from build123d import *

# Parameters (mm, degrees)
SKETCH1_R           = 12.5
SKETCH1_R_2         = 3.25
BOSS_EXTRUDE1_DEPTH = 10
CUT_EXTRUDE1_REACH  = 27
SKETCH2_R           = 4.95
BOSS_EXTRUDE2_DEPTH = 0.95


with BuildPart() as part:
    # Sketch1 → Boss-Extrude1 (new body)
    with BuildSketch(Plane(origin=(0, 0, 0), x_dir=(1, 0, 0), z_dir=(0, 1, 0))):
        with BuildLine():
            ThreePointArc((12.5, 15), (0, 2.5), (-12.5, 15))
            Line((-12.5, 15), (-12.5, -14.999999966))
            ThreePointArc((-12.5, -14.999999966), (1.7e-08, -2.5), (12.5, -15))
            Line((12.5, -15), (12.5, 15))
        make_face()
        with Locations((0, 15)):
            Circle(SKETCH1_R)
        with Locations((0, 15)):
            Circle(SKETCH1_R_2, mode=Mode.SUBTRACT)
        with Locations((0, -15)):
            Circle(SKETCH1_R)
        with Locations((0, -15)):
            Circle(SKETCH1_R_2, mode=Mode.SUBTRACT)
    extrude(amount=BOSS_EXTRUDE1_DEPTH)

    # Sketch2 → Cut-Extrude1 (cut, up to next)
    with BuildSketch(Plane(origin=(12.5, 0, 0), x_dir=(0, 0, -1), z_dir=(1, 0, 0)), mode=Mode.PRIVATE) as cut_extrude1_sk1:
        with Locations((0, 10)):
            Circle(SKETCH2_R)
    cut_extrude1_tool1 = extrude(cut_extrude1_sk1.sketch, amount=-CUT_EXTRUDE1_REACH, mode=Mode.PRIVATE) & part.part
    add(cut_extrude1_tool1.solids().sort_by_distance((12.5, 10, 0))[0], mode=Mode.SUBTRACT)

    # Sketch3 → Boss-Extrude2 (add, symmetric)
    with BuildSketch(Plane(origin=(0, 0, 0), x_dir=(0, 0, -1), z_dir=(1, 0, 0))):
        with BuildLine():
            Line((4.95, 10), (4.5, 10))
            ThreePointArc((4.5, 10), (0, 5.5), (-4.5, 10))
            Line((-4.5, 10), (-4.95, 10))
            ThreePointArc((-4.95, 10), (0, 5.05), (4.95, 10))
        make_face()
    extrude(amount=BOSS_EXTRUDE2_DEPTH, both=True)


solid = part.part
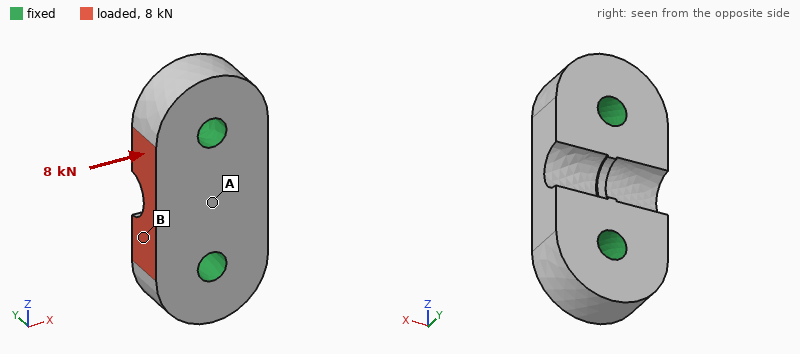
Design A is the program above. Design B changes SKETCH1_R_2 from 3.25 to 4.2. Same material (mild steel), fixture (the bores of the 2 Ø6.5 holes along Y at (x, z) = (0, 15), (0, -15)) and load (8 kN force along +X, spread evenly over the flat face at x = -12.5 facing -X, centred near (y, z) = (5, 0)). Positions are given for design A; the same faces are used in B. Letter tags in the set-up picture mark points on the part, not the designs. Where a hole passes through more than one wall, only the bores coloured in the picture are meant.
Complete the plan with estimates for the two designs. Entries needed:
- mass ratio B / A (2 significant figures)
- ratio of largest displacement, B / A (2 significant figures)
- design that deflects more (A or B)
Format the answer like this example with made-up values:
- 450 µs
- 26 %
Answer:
- 0.96
- 0.86
- A
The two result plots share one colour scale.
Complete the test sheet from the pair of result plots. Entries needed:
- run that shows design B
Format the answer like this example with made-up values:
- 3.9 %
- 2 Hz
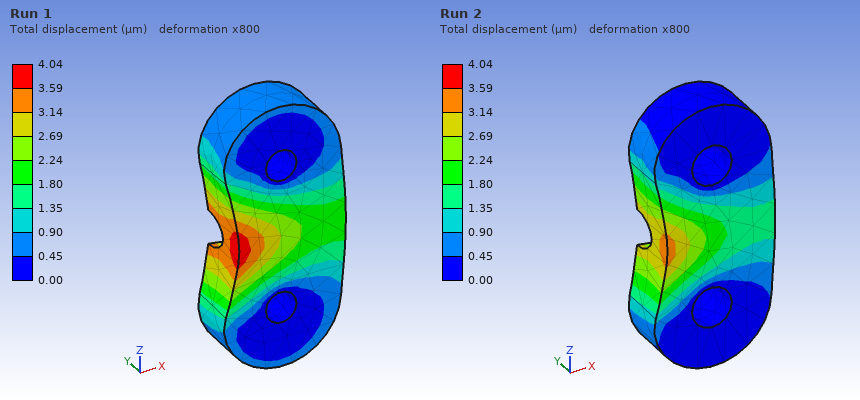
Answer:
- Run 2
